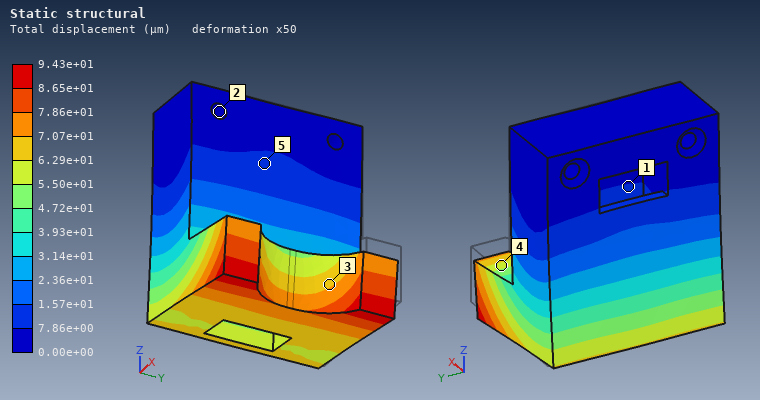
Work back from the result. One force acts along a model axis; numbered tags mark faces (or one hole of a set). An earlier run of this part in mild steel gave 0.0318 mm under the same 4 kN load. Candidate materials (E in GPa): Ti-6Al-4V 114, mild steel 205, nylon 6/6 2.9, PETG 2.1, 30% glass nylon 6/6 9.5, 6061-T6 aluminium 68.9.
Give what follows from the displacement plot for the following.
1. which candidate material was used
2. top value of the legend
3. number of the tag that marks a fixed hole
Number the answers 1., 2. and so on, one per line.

1. 6061-T6 aluminium
2. 9.43e+01 µm
3. 2
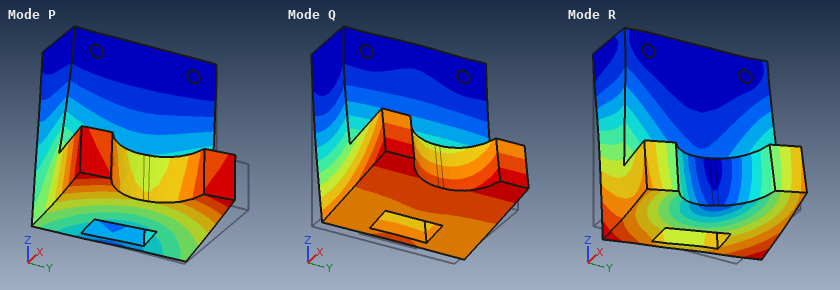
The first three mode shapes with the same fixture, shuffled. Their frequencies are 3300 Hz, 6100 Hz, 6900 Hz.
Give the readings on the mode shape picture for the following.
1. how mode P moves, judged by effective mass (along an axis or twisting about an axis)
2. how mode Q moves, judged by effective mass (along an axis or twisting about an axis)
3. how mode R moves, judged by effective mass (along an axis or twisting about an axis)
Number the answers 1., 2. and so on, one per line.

1. along Y
2. along X
3. along Y
